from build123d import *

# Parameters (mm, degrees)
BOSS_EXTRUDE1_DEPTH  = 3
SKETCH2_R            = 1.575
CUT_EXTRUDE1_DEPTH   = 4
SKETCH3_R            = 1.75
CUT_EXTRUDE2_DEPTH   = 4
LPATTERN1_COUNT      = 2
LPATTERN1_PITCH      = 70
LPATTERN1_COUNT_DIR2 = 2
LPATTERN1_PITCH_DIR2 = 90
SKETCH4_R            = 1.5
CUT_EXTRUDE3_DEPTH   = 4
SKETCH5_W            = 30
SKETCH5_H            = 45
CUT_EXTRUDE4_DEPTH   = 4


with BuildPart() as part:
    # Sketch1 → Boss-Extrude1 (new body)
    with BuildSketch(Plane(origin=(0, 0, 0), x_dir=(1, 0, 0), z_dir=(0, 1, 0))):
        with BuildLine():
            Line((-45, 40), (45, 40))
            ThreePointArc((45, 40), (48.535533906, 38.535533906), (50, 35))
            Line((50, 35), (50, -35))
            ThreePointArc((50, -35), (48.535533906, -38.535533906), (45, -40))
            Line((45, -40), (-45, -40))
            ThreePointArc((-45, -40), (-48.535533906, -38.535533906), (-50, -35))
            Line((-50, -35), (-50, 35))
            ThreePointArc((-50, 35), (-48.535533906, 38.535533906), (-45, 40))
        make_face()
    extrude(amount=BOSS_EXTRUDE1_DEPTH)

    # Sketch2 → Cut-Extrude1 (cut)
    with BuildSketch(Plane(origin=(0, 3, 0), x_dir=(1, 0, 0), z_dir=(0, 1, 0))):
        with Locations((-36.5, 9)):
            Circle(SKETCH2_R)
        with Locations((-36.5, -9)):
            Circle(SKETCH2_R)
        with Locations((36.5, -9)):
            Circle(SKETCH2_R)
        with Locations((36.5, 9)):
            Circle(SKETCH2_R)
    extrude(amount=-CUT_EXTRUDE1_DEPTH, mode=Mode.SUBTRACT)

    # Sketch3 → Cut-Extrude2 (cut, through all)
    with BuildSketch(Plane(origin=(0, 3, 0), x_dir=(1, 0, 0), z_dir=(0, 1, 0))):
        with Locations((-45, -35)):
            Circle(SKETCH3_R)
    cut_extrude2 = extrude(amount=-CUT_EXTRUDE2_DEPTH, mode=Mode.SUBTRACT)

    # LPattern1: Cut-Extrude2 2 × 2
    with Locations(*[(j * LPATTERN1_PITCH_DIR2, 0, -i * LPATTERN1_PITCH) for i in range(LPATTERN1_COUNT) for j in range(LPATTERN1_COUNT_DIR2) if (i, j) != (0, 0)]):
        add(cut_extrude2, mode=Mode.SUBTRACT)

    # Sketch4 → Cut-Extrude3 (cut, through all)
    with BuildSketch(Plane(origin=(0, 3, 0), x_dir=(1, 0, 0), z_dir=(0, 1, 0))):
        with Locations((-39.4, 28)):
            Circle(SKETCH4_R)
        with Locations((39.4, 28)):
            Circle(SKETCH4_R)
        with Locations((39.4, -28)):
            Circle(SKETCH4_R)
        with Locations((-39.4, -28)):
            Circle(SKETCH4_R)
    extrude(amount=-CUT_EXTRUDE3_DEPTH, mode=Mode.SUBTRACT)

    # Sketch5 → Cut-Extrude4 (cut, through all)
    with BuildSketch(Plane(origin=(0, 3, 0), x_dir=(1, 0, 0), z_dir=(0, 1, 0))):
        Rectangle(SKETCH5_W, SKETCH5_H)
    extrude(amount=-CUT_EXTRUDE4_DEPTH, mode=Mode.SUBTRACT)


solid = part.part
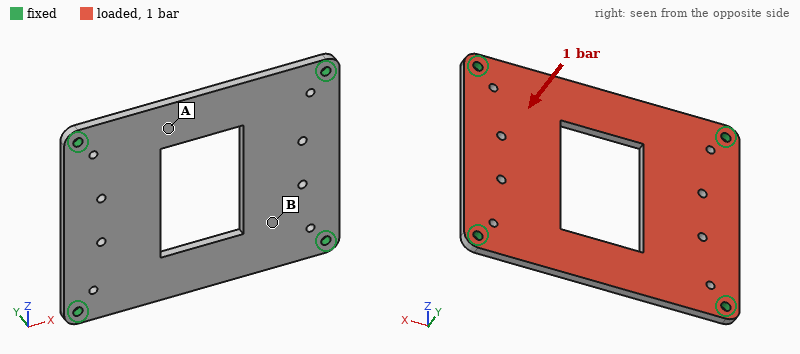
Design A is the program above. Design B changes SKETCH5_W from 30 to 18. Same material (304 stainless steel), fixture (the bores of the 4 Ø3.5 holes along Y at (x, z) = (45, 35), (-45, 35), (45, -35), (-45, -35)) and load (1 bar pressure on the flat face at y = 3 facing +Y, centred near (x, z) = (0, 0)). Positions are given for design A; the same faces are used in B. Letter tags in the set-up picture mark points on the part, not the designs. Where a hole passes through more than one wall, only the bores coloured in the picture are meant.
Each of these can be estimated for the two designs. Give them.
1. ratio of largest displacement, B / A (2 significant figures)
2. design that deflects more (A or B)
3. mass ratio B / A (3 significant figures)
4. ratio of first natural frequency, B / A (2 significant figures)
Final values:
1.3
B
1.08
0.91
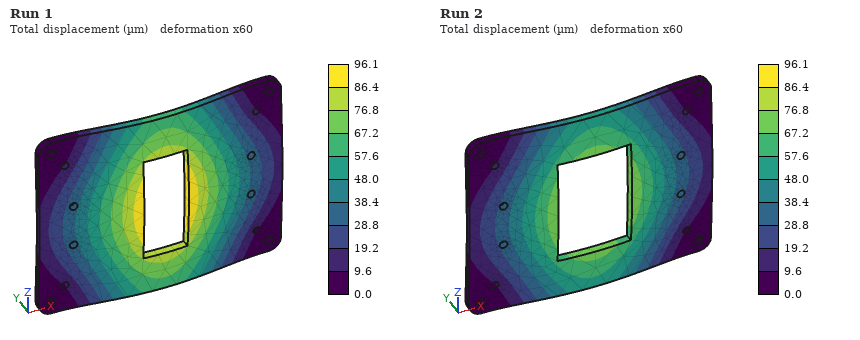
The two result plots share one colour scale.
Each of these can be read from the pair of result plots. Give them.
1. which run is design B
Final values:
Run 1
